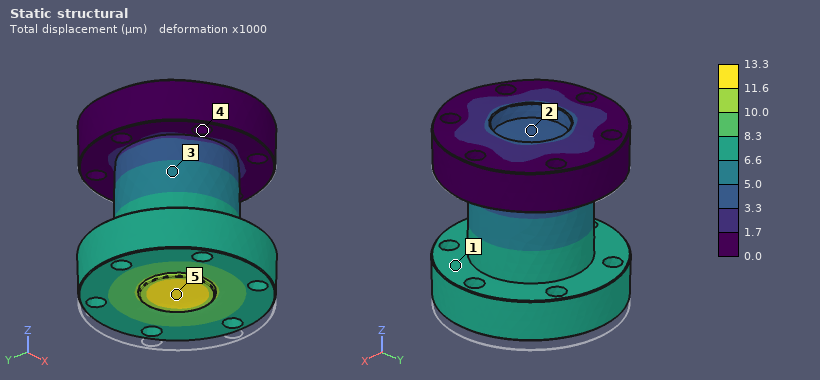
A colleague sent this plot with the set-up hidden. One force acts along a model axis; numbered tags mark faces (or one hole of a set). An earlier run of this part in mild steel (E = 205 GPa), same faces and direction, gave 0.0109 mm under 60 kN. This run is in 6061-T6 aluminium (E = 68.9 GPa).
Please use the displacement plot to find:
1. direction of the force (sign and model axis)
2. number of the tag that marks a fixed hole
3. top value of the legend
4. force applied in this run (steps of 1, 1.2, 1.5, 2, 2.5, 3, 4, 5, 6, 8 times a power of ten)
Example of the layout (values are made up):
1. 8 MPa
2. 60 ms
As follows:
1. +Z
2. 4
3. 13.3 µm
4. 25 kN
